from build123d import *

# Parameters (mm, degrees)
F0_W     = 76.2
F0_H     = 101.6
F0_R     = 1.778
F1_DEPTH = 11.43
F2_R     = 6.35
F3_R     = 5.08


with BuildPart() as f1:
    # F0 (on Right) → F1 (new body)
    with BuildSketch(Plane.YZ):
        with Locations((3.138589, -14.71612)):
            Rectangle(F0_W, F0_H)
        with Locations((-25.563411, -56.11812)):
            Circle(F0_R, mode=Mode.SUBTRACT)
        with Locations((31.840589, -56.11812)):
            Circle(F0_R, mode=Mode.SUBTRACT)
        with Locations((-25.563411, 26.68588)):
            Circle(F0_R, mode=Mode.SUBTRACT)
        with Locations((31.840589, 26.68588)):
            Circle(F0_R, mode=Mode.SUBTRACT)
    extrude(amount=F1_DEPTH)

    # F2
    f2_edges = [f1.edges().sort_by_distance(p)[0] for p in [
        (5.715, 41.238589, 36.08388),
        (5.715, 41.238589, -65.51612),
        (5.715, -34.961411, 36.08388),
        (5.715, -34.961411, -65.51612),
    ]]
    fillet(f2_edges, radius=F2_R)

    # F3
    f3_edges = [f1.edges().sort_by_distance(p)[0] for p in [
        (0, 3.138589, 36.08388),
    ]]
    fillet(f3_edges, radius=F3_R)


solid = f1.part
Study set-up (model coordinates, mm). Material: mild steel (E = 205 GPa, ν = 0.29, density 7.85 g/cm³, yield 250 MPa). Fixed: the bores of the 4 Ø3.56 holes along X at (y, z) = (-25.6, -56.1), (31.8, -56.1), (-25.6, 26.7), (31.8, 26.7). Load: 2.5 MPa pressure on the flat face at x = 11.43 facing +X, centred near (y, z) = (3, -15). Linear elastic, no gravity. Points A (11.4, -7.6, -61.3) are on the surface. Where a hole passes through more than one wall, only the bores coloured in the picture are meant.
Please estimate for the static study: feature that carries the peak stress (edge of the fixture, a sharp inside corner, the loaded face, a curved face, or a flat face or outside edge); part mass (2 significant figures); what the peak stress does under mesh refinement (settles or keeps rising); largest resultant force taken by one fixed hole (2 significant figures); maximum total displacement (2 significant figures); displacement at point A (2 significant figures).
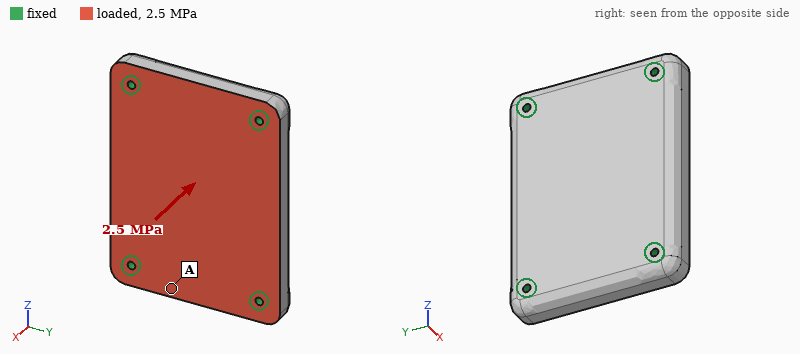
edge of the fixture
670 g
keeps rising
4.8 kN
27 µm
5.2 µm
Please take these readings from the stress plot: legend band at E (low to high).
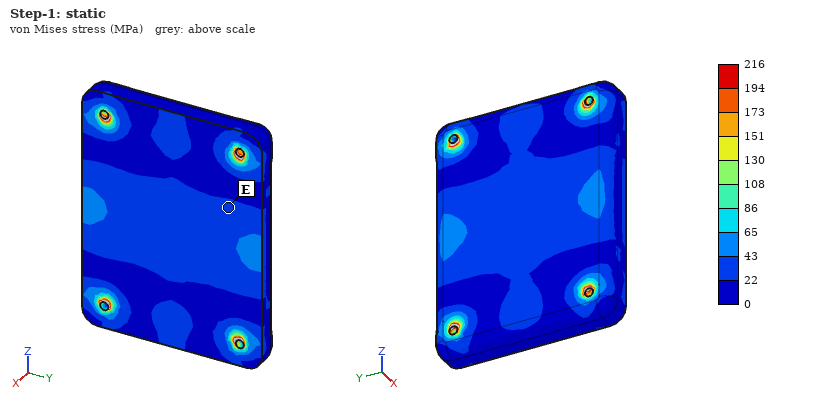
22 to 43 MPa
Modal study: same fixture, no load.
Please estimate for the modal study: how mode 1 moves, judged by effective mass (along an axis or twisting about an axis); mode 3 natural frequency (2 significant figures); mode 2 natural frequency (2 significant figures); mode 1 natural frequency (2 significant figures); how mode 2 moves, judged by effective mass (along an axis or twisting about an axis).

along X
13 kHz
8700 Hz
5900 Hz
twisting about Z
